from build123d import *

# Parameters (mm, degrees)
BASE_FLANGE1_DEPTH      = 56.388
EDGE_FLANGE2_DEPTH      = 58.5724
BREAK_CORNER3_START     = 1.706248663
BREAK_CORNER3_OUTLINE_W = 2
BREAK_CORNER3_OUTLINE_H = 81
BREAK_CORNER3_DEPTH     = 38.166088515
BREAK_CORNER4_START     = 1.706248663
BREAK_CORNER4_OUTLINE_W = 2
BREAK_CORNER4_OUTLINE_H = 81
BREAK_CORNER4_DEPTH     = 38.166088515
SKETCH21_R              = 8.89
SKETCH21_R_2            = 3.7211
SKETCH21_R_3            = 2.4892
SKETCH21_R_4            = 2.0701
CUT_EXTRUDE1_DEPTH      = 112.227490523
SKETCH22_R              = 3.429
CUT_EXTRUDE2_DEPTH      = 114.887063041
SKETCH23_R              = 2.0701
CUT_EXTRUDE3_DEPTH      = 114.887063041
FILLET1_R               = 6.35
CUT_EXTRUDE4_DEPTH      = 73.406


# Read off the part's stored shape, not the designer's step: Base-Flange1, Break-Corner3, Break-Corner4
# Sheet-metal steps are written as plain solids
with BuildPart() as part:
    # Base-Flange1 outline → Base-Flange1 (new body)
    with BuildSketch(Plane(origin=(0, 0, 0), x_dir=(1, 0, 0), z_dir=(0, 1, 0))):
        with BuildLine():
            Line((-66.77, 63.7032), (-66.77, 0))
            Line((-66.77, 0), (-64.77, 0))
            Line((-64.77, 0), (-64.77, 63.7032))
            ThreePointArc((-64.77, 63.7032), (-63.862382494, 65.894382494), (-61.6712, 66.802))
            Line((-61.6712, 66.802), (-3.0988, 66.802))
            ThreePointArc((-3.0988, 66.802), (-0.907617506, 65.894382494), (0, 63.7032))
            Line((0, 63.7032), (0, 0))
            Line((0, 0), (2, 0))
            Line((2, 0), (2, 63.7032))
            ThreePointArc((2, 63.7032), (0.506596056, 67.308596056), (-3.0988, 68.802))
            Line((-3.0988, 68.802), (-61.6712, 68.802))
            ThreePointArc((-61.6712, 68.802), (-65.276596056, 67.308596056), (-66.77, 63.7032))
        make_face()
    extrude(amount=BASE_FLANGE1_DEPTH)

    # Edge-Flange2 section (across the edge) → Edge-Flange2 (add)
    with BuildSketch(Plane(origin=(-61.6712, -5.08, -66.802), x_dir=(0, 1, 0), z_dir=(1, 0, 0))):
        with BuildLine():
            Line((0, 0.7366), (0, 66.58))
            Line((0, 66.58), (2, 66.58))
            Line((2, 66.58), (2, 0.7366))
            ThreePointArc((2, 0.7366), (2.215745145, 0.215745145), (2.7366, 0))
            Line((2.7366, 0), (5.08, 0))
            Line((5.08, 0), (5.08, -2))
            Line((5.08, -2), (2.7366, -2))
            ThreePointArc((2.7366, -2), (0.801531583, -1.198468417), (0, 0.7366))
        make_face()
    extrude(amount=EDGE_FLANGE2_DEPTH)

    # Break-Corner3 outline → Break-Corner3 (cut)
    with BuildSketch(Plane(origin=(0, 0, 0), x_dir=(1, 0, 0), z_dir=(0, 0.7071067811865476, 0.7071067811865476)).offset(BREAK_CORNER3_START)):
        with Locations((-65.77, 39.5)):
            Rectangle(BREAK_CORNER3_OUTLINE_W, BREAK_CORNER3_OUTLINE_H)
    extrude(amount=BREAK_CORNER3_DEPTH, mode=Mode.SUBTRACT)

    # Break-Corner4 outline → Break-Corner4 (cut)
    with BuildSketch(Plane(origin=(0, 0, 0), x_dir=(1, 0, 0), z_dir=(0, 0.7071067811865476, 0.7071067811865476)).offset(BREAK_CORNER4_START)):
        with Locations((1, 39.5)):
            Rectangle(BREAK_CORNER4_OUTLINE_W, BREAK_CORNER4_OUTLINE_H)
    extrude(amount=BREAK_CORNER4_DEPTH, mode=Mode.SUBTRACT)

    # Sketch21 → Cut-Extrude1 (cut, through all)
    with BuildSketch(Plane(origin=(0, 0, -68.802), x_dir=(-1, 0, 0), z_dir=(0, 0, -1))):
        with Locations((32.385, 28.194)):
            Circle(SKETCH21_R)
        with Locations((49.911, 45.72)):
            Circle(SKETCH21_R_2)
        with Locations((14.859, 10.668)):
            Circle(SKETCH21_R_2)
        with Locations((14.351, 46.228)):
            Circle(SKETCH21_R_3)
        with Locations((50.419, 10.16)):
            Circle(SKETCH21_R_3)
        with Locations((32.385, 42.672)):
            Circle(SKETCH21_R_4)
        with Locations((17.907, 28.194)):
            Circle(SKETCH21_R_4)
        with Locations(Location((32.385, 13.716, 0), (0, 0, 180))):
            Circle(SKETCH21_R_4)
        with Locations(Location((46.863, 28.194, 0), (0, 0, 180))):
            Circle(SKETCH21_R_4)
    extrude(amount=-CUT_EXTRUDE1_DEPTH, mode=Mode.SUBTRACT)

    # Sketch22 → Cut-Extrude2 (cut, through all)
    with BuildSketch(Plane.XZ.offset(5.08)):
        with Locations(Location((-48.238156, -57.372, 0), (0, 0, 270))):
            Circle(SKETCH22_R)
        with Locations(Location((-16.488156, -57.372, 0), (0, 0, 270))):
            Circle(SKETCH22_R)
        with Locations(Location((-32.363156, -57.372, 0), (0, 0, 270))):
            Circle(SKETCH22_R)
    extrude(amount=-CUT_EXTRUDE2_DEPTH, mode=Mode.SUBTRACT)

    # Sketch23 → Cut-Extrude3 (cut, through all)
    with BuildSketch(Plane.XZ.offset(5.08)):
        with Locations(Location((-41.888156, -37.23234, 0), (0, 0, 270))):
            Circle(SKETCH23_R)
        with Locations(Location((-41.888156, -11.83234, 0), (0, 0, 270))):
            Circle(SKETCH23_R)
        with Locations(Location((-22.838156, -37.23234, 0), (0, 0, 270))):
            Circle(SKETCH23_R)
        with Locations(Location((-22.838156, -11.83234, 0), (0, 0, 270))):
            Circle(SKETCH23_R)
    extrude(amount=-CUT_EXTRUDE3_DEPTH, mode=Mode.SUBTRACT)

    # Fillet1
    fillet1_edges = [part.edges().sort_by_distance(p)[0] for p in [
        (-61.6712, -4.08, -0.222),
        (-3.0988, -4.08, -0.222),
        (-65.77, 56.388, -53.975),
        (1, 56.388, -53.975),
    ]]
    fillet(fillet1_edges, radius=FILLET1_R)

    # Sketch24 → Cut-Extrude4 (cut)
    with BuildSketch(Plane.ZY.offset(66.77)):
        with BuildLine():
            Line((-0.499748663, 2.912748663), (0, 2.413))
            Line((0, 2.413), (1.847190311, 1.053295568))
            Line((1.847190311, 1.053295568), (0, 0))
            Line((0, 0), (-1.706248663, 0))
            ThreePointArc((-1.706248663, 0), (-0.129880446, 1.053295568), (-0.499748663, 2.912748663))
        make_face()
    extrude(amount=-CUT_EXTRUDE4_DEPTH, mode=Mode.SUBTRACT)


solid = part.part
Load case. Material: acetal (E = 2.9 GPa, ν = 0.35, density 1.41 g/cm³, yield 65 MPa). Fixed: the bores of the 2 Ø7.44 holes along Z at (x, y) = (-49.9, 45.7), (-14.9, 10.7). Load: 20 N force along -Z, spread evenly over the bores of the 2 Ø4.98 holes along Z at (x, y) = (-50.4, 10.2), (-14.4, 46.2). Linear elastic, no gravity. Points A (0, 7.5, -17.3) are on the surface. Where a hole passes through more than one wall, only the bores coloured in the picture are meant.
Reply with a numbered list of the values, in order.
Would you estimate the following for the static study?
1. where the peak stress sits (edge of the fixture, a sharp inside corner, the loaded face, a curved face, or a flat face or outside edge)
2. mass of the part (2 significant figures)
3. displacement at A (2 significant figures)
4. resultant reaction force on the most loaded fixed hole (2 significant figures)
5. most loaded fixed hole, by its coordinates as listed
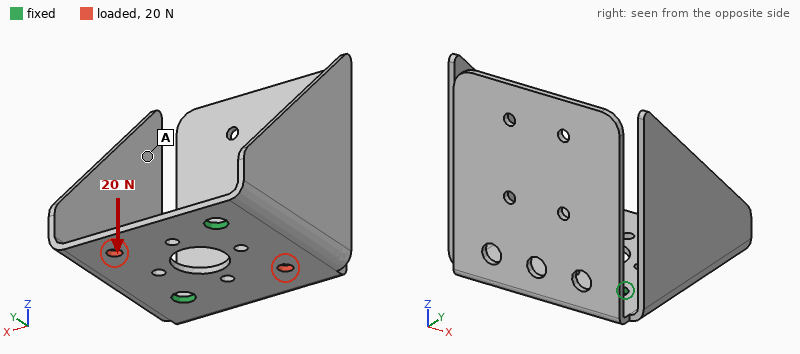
1. a flat face or outside edge
2. 33 g
3. 0.86 mm
4. 11 N
5. (-14.9, 10.7)
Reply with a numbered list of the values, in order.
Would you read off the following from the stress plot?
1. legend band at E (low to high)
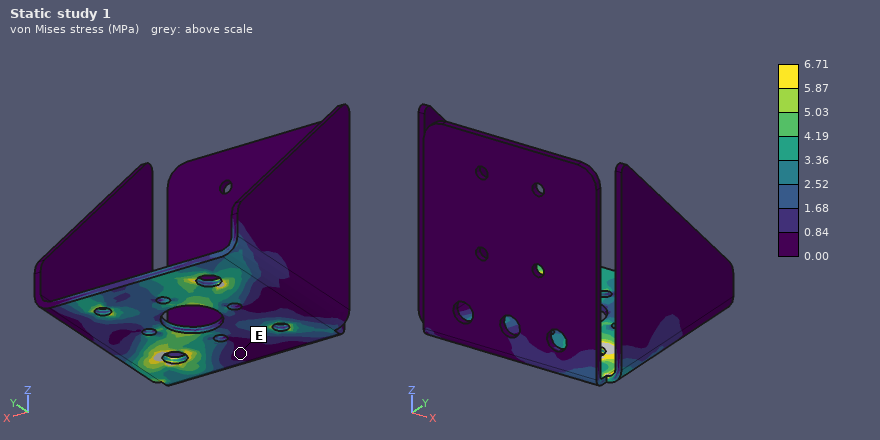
1. 0.00 to 0.84 MPa
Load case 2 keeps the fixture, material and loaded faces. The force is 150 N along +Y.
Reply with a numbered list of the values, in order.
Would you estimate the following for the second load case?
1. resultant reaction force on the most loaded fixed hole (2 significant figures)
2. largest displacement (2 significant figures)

1. 78 N
2. 27 µm
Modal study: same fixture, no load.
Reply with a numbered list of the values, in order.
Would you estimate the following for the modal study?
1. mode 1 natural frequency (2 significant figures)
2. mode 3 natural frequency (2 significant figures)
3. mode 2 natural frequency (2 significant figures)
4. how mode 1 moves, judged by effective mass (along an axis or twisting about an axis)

1. 75 Hz
2. 120 Hz
3. 120 Hz
4. along Y
